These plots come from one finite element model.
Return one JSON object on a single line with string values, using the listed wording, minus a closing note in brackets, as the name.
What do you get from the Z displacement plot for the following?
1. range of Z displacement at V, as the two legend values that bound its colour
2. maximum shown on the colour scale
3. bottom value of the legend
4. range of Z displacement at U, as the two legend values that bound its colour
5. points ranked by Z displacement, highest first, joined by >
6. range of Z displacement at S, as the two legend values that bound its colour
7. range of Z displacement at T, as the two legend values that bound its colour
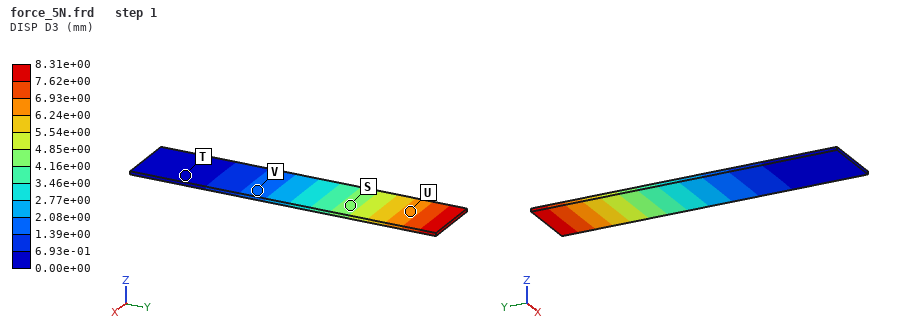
{"range of Z displacement at V, as the two legend values that bound its colour": "1.39e+00 to 2.08e+00 mm", "maximum shown on the colour scale": "8.31e+00 mm", "bottom value of the legend": "0.00e+00 mm", "range of Z displacement at U, as the two legend values that bound its colour": "6.24e+00 to 6.93e+00 mm", "points ranked by Z displacement, highest first, joined by >": "U > S > V > T", "range of Z displacement at S, as the two legend values that bound its colour": "4.16e+00 to 4.85e+00 mm", "range of Z displacement at T, as the two legend values that bound its colour": "0.00e+00 to 6.93e-01 mm"}
